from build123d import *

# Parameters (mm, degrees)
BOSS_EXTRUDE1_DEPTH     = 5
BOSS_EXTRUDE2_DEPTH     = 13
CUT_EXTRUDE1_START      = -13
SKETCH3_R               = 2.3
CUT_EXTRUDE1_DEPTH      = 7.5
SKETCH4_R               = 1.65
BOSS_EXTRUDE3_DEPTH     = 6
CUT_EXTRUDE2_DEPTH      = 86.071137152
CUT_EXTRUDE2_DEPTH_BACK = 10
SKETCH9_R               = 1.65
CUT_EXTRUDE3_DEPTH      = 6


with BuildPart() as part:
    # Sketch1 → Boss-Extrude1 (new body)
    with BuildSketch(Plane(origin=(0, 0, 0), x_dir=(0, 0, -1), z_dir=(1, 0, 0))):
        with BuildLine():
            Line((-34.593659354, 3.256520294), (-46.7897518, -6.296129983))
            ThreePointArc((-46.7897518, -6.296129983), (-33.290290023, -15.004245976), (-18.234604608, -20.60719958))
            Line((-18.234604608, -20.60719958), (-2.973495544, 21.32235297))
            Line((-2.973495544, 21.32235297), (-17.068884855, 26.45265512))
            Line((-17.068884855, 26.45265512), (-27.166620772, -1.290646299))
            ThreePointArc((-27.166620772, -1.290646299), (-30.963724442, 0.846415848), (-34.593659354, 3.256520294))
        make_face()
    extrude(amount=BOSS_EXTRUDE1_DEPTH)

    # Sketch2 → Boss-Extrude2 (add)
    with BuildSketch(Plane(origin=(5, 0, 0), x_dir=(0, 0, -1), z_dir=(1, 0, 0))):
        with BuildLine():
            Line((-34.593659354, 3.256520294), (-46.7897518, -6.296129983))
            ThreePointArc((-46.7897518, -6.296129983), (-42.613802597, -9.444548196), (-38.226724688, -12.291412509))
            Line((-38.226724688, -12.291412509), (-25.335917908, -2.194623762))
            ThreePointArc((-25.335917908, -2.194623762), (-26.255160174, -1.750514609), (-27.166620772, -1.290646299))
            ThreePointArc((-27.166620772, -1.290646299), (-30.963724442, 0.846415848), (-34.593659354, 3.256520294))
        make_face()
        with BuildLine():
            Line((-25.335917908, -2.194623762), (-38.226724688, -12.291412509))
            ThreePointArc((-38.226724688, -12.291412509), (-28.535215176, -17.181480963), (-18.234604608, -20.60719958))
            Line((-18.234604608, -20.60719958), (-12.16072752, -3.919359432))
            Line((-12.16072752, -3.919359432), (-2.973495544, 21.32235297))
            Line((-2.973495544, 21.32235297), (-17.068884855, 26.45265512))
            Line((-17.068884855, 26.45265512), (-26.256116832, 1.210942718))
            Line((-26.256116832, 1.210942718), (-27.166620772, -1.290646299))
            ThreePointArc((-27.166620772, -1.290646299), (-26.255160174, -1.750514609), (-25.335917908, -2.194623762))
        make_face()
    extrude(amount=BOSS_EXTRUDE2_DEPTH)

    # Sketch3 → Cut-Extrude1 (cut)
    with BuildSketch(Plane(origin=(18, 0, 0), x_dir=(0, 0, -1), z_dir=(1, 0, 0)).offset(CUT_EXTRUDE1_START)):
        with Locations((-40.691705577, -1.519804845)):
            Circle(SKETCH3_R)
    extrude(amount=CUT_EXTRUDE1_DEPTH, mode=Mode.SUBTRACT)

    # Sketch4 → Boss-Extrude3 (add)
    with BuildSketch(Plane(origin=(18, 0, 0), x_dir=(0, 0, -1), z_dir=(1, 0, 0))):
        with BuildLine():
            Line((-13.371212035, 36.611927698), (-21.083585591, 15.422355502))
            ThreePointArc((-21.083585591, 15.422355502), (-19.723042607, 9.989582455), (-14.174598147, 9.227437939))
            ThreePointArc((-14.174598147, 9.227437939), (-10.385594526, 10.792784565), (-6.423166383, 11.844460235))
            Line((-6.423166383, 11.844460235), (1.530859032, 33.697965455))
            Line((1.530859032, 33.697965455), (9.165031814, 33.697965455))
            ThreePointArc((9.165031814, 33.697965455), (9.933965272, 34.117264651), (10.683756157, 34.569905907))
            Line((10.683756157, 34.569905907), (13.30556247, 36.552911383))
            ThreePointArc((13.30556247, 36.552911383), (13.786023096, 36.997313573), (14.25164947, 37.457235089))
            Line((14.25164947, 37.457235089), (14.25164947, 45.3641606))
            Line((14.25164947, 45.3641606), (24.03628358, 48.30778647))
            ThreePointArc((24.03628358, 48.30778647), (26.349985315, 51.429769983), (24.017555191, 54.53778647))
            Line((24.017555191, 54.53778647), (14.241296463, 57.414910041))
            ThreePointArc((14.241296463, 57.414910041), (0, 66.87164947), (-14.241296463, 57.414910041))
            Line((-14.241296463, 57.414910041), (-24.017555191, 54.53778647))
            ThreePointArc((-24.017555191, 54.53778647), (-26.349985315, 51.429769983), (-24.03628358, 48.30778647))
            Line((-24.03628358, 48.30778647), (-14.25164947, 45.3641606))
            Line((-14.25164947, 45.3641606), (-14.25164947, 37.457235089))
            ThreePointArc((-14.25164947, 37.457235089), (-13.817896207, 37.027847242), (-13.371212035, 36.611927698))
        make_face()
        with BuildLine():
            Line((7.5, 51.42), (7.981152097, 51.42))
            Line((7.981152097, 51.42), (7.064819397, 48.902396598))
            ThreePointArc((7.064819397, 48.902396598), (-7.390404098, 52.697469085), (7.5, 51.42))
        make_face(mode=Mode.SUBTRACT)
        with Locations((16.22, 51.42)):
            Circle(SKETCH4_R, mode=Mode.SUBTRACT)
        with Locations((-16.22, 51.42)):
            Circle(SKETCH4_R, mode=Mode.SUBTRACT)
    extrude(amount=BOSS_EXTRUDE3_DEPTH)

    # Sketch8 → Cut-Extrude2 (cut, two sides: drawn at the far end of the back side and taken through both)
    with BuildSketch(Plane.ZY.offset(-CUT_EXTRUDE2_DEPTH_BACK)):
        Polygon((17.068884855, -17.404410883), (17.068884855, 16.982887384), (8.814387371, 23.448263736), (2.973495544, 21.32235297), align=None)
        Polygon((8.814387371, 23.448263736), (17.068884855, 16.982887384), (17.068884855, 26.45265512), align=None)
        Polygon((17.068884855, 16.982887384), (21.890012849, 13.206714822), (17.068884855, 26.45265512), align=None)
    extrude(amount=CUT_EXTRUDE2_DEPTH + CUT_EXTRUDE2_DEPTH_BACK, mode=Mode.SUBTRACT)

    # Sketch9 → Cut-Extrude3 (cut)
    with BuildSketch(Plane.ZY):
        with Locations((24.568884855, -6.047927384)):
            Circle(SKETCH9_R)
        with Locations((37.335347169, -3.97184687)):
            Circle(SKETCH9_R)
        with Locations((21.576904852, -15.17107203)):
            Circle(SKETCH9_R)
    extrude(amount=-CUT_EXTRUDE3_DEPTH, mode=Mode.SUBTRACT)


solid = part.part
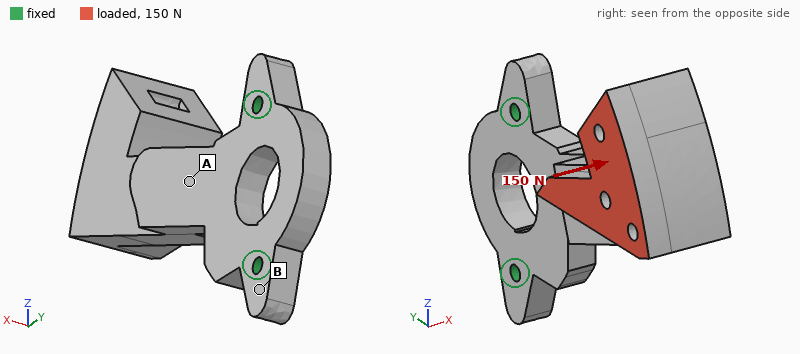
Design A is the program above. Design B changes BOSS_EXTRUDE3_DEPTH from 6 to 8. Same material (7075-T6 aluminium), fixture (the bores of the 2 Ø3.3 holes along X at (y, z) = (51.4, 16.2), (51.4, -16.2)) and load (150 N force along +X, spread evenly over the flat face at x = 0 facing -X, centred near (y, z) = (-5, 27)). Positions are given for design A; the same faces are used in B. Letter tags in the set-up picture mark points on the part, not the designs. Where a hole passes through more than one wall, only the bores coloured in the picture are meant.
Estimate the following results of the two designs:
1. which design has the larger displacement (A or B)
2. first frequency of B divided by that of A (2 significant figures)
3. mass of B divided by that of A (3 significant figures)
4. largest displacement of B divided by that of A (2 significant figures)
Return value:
A
1.5
1.13
0.47
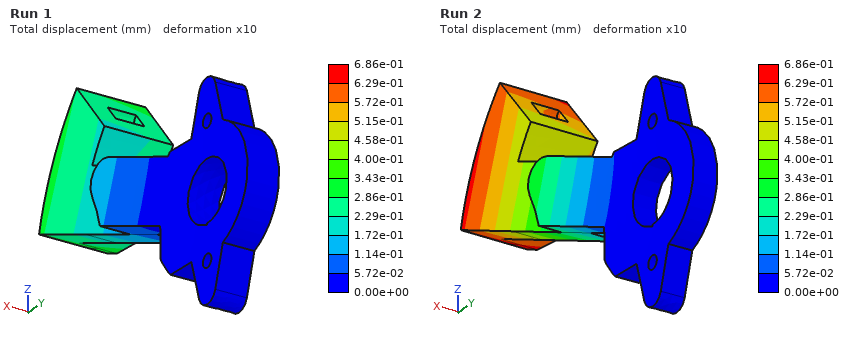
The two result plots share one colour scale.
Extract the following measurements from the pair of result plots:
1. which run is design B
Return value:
Run 1
